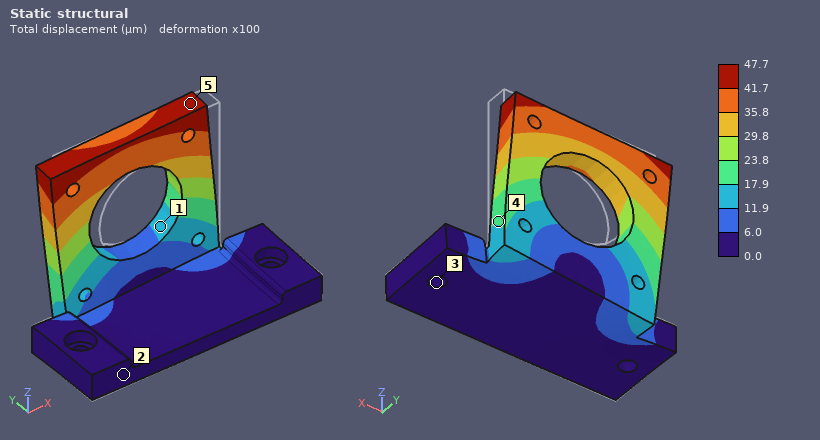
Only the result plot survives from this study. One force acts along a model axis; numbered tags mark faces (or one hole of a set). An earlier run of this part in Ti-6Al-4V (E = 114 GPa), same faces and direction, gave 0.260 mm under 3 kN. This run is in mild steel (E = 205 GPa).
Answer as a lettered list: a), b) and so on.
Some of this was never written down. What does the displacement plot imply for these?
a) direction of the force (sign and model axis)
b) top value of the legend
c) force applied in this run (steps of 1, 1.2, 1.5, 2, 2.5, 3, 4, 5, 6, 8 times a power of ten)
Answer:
a) -X
b) 47.7 µm
c) 1 kN
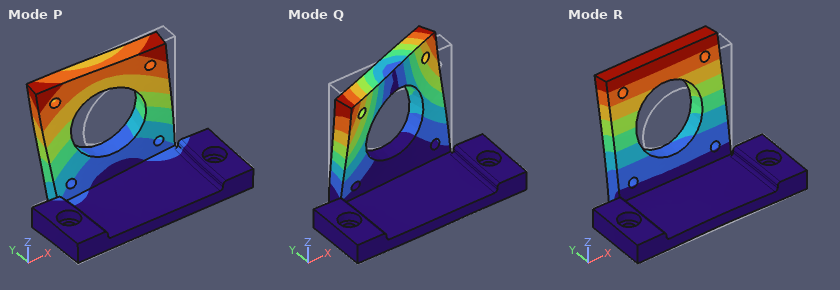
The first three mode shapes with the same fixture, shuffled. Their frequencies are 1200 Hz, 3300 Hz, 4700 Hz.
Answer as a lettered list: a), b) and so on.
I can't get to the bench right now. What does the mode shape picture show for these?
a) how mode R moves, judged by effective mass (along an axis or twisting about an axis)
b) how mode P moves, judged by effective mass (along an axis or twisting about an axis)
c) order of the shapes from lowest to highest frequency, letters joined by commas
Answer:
a) along Y
b) along X
c) R, P, Q
